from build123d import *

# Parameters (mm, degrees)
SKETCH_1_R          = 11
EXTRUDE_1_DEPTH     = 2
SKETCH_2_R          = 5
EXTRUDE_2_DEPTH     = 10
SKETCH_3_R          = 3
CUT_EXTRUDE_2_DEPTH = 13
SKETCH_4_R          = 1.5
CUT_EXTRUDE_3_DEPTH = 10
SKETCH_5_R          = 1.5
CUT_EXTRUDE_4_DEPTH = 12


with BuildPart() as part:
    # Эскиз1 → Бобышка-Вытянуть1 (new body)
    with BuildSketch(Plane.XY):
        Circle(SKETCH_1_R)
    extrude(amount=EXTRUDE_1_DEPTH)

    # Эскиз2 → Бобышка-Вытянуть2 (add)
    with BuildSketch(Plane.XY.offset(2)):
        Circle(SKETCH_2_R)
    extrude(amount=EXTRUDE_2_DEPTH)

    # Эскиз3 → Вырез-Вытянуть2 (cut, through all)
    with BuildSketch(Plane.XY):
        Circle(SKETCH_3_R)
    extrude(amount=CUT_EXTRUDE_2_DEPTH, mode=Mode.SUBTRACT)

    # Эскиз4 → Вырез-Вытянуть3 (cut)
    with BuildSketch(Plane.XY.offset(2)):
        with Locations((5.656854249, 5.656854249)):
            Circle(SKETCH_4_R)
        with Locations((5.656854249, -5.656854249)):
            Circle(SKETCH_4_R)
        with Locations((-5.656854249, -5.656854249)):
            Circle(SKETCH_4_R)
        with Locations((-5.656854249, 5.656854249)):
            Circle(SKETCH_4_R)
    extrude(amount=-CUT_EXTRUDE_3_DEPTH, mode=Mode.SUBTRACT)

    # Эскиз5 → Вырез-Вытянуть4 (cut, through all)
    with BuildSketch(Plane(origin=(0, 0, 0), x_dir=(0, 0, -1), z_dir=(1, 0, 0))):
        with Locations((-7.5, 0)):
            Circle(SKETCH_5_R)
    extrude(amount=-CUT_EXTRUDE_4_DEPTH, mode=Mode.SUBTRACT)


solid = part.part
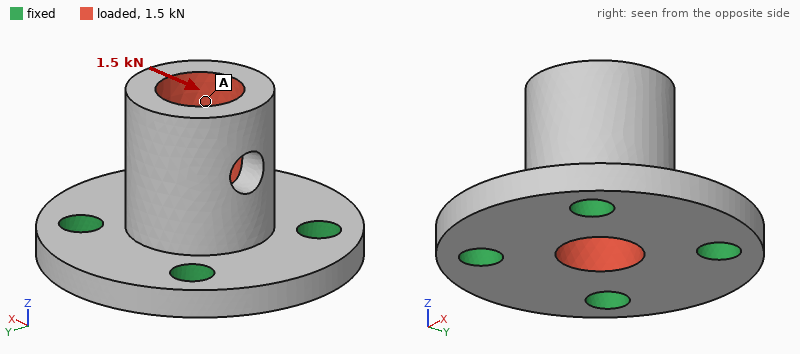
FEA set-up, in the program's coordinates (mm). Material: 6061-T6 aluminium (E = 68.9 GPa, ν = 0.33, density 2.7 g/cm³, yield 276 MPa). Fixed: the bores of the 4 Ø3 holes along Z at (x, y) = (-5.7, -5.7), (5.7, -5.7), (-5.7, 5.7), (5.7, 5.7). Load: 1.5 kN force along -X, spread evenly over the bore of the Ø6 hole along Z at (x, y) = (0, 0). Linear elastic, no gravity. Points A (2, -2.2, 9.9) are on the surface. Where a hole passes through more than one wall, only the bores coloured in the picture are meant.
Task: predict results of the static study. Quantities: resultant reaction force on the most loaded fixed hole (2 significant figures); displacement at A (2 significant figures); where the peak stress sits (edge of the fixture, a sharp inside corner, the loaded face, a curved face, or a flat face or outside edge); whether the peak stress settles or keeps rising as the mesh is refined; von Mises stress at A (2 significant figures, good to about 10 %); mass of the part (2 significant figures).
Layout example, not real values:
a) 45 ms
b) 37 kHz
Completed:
a) 560 N
b) 27 µm
c) edge of the fixture
d) keeps rising
e) 23 MPa
f) 3.1 g
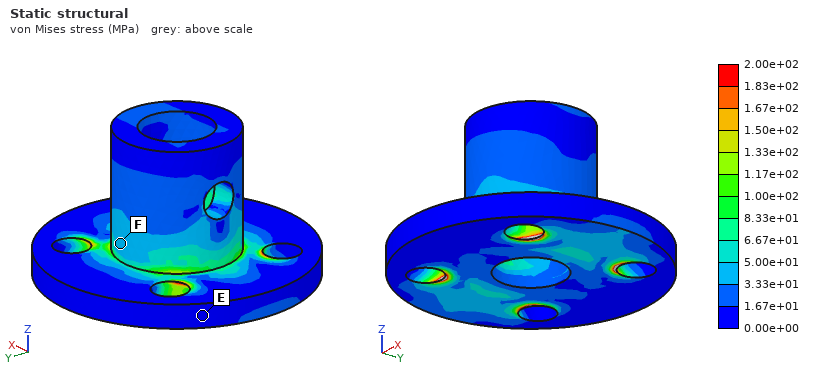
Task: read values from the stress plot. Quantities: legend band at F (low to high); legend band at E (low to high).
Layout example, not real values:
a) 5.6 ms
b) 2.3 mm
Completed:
a) 3.33e+01 to 5.00e+01 MPa
b) 0.00e+00 to 1.67e+01 MPa
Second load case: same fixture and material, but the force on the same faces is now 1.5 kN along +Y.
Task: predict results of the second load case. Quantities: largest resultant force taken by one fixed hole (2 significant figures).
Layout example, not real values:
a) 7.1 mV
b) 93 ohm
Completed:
a) 570 N
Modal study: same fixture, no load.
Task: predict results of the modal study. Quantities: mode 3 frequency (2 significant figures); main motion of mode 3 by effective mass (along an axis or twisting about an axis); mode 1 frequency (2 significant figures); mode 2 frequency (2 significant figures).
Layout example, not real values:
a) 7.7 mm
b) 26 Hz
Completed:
a) 53 kHz
b) along Z
c) 30 kHz
d) 31 kHz
